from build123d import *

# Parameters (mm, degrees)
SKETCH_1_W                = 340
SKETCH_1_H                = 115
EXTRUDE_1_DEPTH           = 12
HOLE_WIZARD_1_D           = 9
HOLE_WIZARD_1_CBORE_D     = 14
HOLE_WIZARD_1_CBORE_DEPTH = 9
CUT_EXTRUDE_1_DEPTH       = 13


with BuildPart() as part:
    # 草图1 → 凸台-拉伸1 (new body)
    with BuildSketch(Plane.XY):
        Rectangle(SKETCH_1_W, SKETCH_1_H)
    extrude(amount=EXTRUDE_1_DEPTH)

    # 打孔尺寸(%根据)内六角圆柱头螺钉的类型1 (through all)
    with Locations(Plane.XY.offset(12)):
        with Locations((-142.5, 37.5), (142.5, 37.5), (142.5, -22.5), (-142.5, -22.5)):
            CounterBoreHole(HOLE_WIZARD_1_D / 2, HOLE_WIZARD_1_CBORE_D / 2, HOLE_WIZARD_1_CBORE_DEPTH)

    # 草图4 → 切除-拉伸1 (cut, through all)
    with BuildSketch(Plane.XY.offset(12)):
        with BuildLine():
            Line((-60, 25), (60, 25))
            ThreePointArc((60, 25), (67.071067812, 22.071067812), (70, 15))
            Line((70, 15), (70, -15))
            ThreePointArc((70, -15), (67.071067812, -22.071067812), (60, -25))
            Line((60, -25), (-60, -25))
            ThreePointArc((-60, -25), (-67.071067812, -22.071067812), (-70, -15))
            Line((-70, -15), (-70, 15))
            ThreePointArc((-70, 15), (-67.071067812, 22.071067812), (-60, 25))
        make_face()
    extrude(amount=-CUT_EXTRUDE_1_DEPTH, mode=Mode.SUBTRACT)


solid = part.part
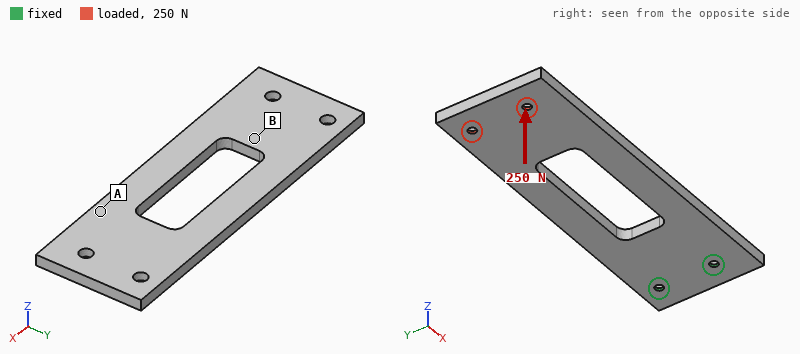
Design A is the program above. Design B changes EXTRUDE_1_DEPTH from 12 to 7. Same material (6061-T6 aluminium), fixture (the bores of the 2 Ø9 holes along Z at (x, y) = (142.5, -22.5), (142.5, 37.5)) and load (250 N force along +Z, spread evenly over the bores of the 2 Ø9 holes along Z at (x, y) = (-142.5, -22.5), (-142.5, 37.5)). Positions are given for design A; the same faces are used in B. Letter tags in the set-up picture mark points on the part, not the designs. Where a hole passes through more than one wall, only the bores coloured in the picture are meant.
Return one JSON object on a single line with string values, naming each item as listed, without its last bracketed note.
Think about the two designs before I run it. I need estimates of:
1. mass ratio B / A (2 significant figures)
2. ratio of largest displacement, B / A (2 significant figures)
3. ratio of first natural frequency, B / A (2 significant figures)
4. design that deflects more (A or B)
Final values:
{"mass ratio B / A": "0.58", "ratio of largest displacement, B / A": "3.8", "ratio of first natural frequency, B / A": "0.70", "design that deflects more": "B"}
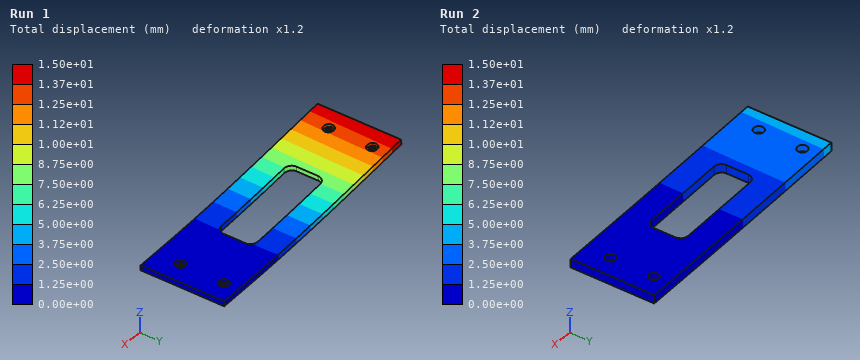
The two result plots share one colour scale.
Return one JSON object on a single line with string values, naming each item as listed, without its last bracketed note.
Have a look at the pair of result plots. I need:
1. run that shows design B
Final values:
{"run that shows design B": "Run 1"}
